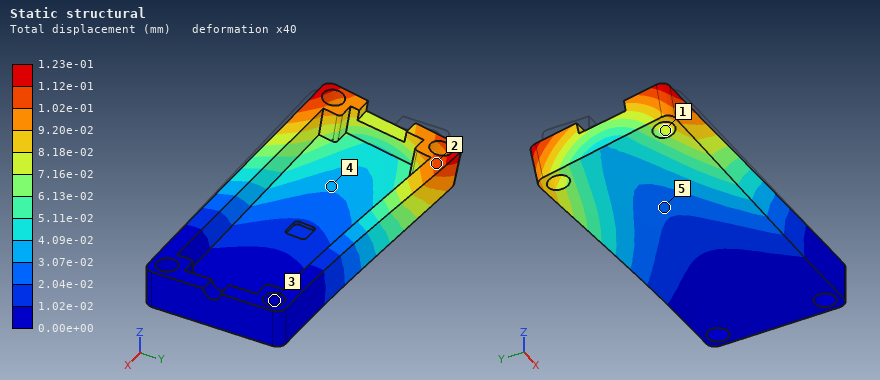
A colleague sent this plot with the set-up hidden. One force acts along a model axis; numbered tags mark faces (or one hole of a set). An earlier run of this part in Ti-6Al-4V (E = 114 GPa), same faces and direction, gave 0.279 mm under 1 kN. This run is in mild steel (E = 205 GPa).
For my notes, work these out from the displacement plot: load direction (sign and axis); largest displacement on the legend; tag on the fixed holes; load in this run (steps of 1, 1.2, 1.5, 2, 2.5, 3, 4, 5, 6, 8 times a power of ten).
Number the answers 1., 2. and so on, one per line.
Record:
1. +Y
2. 1.23e-01 mm
3. 3
4. 800 N
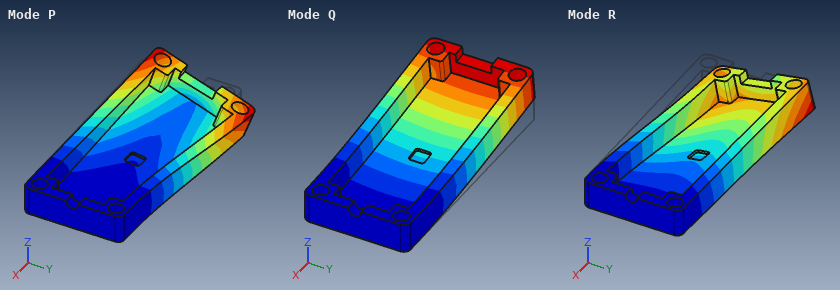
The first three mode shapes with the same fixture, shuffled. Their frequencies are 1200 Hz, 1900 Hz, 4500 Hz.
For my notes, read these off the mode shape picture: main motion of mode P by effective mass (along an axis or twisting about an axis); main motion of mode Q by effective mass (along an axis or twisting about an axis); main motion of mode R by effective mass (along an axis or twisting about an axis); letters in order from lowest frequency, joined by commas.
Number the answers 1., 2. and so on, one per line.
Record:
1. along Y
2. along Z
3. along Y
4. Q, P, R
